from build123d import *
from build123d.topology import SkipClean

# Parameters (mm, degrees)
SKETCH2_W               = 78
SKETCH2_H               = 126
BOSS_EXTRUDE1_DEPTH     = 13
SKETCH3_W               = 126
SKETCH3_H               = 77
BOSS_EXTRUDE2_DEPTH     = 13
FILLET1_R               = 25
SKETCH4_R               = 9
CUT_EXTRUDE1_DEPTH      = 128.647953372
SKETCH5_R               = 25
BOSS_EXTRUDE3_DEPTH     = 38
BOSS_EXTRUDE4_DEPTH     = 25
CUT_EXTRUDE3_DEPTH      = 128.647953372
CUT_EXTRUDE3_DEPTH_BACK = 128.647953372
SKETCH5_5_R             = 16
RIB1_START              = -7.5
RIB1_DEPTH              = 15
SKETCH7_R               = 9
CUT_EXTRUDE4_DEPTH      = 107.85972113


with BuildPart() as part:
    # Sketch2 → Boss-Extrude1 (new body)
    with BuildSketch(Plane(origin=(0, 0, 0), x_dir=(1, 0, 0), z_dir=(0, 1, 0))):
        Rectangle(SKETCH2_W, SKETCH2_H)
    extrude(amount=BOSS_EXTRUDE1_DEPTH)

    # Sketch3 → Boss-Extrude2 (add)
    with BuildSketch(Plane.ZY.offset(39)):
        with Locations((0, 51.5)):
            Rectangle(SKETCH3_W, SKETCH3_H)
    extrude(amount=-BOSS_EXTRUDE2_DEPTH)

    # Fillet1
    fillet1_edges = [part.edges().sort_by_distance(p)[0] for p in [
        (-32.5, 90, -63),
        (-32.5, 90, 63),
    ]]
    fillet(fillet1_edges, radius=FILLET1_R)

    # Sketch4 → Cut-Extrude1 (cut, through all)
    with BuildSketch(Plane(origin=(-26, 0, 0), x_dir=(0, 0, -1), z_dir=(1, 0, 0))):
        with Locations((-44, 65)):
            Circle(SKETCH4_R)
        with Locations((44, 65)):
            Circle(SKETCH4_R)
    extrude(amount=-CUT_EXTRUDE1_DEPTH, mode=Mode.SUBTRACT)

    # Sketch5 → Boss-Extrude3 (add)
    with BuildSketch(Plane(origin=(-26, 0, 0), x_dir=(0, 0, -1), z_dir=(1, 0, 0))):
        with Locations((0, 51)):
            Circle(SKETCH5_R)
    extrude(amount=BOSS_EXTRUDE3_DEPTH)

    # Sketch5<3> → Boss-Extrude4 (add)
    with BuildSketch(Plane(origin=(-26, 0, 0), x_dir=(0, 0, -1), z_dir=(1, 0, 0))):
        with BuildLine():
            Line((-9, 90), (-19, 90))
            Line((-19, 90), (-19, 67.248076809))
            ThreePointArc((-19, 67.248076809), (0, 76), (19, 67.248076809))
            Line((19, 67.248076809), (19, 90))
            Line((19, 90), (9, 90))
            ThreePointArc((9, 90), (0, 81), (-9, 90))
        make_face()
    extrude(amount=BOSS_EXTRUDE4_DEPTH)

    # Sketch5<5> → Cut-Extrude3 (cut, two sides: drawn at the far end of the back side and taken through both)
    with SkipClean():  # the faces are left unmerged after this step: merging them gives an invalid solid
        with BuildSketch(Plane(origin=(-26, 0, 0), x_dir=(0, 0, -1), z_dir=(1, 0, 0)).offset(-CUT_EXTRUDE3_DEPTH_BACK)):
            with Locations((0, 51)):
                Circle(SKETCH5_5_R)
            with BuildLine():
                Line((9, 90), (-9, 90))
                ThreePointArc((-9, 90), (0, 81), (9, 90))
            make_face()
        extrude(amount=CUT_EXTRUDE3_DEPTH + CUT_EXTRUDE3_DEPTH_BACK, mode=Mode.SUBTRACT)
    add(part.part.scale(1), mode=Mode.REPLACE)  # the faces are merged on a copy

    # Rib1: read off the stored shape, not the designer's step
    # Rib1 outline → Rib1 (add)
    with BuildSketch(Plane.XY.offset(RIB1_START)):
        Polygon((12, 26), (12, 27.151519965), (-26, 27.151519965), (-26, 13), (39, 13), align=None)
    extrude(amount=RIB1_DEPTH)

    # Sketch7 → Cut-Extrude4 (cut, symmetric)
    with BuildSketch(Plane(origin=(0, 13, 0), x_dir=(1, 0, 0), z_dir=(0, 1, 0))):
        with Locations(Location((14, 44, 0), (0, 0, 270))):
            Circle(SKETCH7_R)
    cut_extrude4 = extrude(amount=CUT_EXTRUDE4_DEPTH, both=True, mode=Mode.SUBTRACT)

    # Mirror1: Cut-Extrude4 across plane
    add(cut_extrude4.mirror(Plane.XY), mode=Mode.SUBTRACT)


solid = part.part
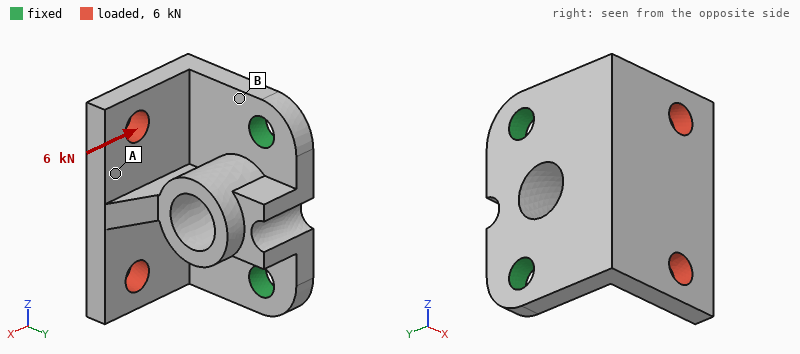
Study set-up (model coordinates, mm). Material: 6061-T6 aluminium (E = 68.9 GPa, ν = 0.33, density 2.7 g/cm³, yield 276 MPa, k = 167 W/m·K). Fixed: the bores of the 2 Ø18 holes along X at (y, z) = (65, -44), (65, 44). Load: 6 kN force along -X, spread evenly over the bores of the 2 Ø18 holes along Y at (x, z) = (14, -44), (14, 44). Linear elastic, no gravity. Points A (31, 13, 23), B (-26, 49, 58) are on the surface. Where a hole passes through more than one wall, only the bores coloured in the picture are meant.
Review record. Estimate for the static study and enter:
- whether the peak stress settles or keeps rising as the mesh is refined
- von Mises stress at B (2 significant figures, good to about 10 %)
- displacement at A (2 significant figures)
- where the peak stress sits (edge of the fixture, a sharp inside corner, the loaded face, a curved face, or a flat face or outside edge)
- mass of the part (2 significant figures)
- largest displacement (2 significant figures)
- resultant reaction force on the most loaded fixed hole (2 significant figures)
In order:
keeps rising
53 MPa
0.22 mm
edge of the fixture
790 g
0.27 mm
3.1 kN
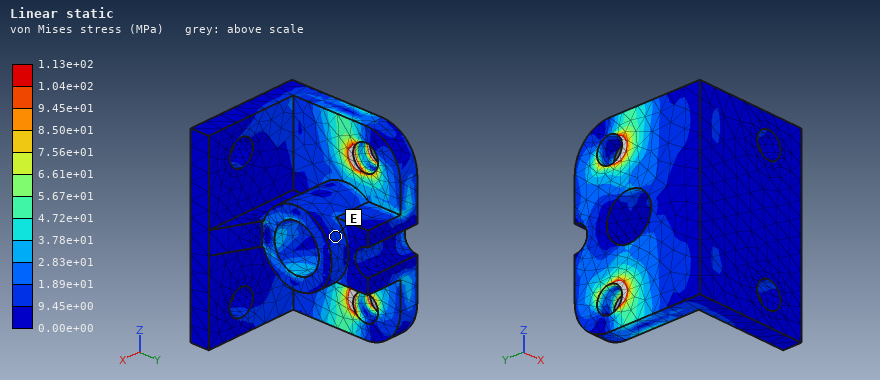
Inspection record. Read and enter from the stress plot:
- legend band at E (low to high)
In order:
9.45e+00 to 1.89e+01 MPa
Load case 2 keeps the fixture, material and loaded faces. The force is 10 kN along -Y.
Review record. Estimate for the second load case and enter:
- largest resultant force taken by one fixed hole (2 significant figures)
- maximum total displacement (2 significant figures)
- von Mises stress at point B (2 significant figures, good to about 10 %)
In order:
5.0 kN
0.60 mm
77 MPa
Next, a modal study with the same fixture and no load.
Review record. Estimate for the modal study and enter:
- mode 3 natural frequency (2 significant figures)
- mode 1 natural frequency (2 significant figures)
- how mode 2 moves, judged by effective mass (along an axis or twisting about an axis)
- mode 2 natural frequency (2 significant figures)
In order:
3400 Hz
1300 Hz
along Z
2500 Hz
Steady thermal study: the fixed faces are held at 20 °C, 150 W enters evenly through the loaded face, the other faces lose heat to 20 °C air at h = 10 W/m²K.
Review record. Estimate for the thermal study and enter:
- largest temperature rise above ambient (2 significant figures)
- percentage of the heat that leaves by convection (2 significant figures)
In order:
53 K
7.8 %
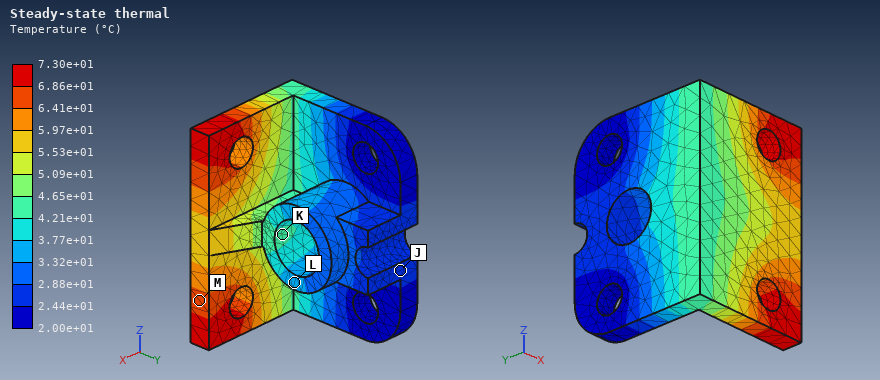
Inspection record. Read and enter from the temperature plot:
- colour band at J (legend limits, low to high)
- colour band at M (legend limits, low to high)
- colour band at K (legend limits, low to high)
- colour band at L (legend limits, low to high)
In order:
2.44e+01 to 2.88e+01 °C
6.41e+01 to 6.86e+01 °C
4.21e+01 to 4.65e+01 °C
3.32e+01 to 3.77e+01 °C
